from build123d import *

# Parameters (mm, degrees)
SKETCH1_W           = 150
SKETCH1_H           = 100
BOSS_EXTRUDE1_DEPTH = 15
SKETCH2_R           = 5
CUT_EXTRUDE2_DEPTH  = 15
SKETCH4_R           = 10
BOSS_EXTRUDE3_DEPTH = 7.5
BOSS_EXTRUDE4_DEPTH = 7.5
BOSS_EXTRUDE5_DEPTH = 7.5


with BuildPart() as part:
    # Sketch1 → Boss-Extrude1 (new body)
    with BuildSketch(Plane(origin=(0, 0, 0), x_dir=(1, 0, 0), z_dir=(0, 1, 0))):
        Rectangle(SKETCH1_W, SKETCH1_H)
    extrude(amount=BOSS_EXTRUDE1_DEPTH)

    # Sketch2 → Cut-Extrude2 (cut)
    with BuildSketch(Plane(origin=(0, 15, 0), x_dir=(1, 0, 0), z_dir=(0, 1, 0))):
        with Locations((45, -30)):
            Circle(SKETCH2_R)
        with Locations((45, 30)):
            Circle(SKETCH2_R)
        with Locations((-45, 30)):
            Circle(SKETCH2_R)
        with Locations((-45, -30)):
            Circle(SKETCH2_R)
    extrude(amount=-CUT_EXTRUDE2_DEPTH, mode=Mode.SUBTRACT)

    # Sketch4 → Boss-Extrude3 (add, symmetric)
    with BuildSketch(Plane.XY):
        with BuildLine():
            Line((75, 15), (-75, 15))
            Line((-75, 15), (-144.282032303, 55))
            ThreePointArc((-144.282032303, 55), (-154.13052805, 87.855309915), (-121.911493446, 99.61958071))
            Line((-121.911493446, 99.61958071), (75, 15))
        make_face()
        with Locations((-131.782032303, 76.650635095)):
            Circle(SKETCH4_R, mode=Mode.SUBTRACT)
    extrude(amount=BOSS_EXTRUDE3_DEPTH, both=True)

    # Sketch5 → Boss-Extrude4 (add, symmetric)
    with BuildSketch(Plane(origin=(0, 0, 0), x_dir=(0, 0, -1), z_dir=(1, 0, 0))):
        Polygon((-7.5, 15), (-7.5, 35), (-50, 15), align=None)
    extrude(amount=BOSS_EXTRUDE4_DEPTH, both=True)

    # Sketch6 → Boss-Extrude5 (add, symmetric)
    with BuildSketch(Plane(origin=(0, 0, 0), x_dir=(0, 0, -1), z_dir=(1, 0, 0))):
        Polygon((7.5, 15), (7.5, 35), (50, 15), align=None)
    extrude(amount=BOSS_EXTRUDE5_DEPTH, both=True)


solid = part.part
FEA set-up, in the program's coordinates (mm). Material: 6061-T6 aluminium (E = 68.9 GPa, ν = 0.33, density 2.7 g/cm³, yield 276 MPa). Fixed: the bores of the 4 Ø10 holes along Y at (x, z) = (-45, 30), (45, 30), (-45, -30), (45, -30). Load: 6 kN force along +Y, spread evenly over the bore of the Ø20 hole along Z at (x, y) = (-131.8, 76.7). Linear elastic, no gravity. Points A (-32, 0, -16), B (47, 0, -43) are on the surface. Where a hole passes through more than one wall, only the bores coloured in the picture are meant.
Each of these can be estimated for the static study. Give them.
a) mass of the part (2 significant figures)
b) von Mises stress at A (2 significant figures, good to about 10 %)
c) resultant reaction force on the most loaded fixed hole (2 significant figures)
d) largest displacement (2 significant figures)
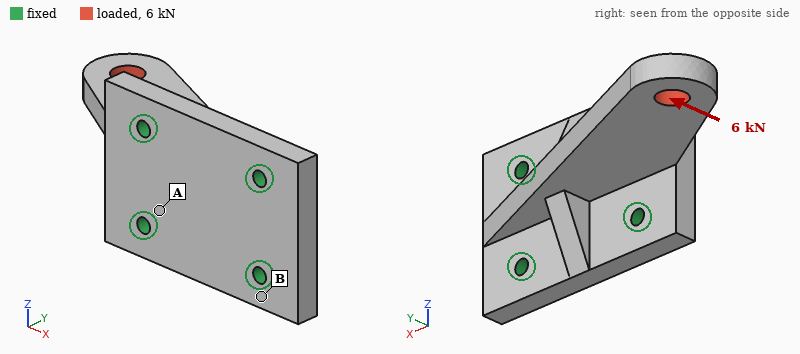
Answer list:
990 g
17 MPa
6.0 kN
0.28 mm
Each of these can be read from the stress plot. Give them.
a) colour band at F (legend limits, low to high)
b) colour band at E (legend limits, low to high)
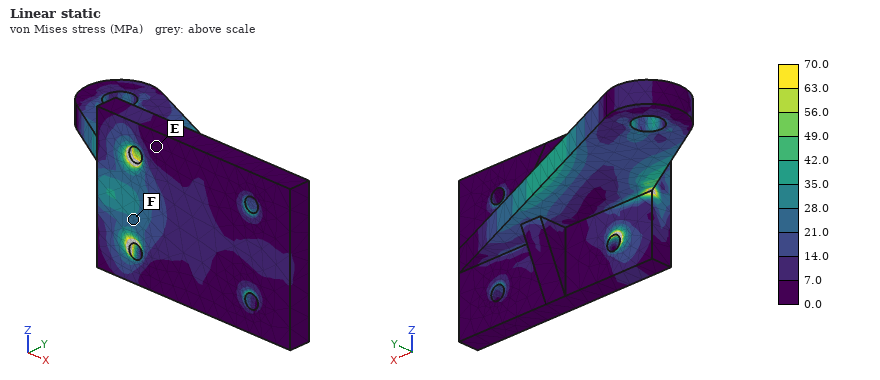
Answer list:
21.0 to 28.0 MPa
0.0 to 7.0 MPa
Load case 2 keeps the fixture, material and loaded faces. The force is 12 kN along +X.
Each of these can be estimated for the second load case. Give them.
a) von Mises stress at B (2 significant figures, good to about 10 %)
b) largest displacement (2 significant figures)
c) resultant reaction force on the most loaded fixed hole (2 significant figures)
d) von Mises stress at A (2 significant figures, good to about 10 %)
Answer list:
9.4 MPa
0.32 mm
6.0 kN
12 MPa
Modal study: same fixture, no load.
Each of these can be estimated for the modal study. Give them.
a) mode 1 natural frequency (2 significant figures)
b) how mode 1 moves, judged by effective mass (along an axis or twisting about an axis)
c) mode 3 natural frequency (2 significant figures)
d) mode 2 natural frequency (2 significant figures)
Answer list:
920 Hz
along Z
3200 Hz
2300 Hz
